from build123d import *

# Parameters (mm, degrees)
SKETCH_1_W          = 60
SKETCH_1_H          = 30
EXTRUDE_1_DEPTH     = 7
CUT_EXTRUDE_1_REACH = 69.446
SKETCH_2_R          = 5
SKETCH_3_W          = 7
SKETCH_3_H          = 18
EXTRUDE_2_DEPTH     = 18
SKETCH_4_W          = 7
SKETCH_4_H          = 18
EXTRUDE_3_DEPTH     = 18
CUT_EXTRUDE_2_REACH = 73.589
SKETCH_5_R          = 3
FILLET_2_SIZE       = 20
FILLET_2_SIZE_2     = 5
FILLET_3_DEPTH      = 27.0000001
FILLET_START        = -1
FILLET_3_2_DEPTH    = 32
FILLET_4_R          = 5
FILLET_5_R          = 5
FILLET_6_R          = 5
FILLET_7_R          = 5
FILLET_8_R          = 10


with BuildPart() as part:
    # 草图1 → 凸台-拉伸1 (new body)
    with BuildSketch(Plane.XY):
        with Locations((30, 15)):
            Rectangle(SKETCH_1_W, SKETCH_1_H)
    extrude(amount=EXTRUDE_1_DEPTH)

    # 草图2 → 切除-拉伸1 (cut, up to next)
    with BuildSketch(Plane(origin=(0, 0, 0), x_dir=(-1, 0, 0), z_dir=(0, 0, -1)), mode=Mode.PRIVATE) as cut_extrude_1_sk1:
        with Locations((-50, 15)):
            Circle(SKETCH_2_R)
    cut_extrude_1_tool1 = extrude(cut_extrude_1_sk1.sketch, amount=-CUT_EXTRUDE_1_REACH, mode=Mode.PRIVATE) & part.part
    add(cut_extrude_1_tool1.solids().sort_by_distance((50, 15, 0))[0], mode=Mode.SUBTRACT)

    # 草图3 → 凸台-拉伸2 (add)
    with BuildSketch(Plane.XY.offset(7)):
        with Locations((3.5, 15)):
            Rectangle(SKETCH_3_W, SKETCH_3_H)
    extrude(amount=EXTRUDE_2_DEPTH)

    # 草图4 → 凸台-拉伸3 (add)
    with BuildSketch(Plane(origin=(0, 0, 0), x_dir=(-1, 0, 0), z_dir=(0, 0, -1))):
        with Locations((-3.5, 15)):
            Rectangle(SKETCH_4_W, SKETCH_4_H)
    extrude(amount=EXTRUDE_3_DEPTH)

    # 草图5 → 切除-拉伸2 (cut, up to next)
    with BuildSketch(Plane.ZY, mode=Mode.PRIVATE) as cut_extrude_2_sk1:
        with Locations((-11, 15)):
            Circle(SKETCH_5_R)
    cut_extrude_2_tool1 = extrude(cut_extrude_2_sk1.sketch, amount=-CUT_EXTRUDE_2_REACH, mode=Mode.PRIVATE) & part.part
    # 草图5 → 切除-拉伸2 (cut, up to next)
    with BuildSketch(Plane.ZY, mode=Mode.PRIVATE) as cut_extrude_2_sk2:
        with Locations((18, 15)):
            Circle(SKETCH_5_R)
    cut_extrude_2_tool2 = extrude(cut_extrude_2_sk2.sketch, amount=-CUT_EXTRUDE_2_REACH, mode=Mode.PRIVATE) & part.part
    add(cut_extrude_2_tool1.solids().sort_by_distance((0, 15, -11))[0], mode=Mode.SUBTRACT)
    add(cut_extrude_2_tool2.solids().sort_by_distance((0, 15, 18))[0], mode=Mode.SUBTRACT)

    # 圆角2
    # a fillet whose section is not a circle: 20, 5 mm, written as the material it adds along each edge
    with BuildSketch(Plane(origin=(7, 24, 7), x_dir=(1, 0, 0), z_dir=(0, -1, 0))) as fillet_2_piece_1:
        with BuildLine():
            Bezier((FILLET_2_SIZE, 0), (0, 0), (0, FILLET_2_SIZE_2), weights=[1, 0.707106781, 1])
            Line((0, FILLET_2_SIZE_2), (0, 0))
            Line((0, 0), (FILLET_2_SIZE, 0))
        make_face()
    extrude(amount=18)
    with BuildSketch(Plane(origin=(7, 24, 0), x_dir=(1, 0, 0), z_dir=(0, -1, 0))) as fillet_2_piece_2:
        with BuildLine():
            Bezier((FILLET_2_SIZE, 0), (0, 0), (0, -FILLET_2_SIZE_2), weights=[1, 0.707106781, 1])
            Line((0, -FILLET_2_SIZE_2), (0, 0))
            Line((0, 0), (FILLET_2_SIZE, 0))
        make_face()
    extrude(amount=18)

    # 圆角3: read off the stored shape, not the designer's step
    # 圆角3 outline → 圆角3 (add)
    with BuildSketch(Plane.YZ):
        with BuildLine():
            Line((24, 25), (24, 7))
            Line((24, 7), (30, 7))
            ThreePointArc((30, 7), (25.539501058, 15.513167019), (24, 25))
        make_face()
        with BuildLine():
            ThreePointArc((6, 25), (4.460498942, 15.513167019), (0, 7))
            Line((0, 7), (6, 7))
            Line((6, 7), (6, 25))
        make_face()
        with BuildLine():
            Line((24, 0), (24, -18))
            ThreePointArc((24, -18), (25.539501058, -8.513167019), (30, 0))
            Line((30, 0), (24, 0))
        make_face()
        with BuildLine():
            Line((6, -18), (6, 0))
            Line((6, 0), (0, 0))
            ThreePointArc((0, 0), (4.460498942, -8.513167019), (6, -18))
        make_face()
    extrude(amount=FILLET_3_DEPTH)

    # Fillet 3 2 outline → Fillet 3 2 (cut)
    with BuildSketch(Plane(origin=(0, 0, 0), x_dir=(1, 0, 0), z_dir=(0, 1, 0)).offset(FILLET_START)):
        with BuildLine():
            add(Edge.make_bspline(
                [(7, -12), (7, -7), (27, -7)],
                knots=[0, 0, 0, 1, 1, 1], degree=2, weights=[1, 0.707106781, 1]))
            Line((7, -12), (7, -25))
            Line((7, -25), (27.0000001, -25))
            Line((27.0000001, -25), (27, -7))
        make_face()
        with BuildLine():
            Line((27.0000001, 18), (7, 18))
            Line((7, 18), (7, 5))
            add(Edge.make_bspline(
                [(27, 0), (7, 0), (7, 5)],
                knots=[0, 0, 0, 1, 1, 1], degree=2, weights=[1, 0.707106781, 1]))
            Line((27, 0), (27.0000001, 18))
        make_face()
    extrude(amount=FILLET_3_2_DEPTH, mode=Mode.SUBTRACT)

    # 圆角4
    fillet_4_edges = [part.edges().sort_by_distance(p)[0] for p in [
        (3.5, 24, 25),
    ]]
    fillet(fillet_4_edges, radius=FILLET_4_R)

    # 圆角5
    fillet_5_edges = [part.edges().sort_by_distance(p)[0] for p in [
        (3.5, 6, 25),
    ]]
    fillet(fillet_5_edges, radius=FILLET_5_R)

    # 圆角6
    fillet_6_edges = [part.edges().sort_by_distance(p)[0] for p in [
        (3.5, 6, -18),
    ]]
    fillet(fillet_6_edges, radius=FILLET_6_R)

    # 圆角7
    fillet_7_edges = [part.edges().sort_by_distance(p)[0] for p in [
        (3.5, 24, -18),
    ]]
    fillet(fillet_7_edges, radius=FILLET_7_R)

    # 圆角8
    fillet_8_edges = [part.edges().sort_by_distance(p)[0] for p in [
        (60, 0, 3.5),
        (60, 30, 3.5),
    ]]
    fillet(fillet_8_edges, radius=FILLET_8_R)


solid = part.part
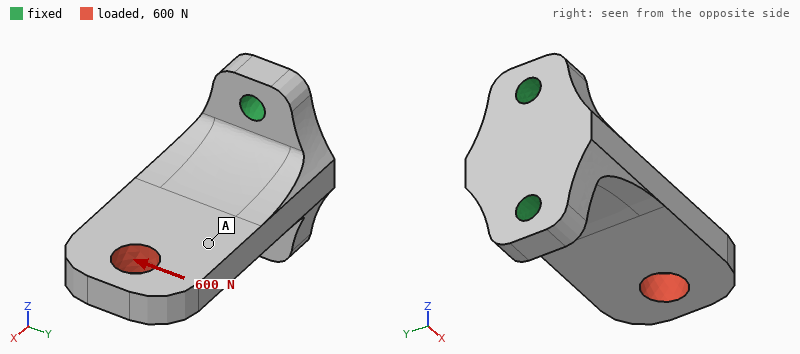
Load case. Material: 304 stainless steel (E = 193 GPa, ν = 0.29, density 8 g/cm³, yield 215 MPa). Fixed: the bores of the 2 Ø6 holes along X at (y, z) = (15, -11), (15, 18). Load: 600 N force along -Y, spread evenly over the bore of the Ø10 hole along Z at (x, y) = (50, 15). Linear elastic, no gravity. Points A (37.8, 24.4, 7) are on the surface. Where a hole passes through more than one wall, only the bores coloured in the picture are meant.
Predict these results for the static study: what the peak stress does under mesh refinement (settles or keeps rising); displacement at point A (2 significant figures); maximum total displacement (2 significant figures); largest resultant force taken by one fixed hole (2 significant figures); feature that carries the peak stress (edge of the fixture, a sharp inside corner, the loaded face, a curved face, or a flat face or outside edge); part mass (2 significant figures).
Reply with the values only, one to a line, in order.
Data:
keeps rising
26 µm
43 µm
300 N
edge of the fixture
140 g
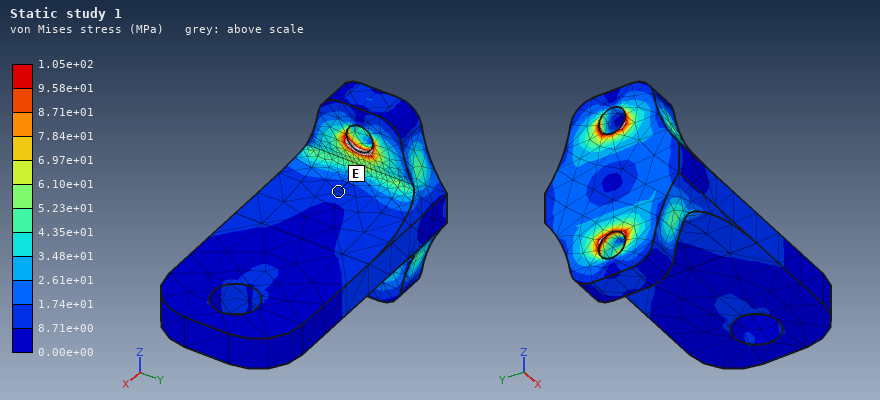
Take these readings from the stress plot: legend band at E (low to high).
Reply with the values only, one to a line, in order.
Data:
8.71e+00 to 1.74e+01 MPa
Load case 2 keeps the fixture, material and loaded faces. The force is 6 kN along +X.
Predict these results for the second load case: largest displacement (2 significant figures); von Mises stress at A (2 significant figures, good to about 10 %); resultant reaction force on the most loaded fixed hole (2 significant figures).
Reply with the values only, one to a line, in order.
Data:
15 µm
31 MPa
3.1 kN
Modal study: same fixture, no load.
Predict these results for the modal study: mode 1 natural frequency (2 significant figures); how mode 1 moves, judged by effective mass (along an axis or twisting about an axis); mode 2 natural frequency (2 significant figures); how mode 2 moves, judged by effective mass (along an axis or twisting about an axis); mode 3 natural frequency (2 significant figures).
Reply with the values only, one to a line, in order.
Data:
2700 Hz
along Z
3200 Hz
along Y
8000 Hz
